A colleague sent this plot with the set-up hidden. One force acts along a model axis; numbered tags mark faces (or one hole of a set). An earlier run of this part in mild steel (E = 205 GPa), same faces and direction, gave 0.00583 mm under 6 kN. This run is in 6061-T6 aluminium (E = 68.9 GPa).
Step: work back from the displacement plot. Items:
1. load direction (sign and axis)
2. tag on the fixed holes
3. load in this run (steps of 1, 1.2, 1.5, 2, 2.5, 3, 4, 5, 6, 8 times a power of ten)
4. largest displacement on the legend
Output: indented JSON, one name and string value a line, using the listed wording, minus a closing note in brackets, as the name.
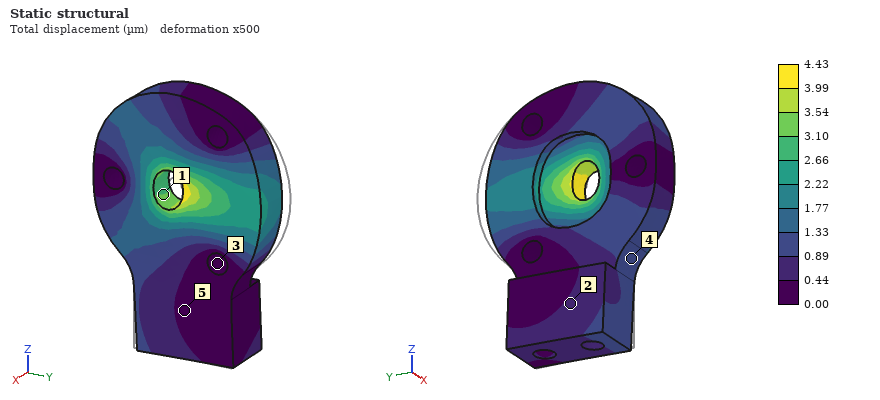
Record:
{
  "load direction": "-Y",
  "tag on the fixed holes": "3",
  "load in this run": "1.5 kN",
  "largest displacement on the legend": "4.43 µm"
}
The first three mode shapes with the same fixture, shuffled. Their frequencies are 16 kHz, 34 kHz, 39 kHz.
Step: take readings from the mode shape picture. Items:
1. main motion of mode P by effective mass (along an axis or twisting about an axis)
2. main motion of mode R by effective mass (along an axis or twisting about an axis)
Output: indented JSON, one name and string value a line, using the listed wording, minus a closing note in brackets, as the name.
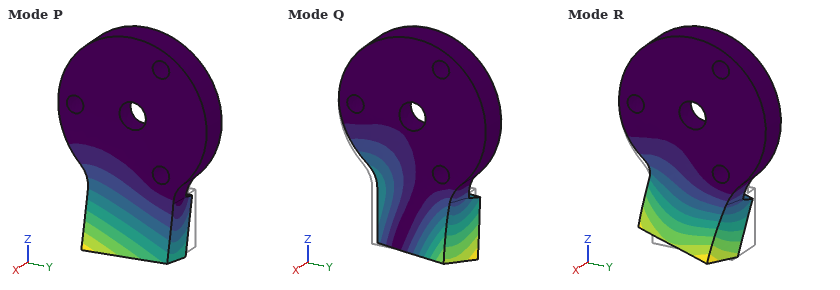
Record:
{
  "main motion of mode P by effective mass": "along X",
  "main motion of mode R by effective mass": "along Y"
}
